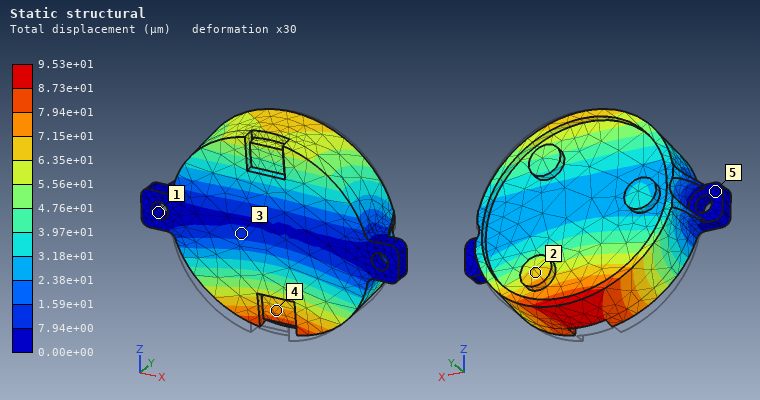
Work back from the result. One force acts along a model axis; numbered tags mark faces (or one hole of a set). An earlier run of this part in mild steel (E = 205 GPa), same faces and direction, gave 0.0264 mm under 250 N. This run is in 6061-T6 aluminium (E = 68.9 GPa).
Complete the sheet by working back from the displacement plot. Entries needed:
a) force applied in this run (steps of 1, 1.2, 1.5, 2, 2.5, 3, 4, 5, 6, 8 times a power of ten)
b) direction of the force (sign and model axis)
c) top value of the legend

300 N
+Y
9.53e+01 µm
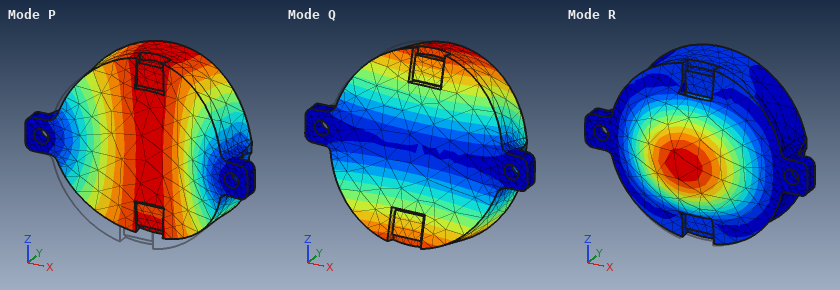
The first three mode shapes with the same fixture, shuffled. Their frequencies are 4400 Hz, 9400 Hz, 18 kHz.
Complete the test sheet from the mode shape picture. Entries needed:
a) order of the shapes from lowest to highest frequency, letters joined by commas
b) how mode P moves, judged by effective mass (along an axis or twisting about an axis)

Q, P, R
along Y
